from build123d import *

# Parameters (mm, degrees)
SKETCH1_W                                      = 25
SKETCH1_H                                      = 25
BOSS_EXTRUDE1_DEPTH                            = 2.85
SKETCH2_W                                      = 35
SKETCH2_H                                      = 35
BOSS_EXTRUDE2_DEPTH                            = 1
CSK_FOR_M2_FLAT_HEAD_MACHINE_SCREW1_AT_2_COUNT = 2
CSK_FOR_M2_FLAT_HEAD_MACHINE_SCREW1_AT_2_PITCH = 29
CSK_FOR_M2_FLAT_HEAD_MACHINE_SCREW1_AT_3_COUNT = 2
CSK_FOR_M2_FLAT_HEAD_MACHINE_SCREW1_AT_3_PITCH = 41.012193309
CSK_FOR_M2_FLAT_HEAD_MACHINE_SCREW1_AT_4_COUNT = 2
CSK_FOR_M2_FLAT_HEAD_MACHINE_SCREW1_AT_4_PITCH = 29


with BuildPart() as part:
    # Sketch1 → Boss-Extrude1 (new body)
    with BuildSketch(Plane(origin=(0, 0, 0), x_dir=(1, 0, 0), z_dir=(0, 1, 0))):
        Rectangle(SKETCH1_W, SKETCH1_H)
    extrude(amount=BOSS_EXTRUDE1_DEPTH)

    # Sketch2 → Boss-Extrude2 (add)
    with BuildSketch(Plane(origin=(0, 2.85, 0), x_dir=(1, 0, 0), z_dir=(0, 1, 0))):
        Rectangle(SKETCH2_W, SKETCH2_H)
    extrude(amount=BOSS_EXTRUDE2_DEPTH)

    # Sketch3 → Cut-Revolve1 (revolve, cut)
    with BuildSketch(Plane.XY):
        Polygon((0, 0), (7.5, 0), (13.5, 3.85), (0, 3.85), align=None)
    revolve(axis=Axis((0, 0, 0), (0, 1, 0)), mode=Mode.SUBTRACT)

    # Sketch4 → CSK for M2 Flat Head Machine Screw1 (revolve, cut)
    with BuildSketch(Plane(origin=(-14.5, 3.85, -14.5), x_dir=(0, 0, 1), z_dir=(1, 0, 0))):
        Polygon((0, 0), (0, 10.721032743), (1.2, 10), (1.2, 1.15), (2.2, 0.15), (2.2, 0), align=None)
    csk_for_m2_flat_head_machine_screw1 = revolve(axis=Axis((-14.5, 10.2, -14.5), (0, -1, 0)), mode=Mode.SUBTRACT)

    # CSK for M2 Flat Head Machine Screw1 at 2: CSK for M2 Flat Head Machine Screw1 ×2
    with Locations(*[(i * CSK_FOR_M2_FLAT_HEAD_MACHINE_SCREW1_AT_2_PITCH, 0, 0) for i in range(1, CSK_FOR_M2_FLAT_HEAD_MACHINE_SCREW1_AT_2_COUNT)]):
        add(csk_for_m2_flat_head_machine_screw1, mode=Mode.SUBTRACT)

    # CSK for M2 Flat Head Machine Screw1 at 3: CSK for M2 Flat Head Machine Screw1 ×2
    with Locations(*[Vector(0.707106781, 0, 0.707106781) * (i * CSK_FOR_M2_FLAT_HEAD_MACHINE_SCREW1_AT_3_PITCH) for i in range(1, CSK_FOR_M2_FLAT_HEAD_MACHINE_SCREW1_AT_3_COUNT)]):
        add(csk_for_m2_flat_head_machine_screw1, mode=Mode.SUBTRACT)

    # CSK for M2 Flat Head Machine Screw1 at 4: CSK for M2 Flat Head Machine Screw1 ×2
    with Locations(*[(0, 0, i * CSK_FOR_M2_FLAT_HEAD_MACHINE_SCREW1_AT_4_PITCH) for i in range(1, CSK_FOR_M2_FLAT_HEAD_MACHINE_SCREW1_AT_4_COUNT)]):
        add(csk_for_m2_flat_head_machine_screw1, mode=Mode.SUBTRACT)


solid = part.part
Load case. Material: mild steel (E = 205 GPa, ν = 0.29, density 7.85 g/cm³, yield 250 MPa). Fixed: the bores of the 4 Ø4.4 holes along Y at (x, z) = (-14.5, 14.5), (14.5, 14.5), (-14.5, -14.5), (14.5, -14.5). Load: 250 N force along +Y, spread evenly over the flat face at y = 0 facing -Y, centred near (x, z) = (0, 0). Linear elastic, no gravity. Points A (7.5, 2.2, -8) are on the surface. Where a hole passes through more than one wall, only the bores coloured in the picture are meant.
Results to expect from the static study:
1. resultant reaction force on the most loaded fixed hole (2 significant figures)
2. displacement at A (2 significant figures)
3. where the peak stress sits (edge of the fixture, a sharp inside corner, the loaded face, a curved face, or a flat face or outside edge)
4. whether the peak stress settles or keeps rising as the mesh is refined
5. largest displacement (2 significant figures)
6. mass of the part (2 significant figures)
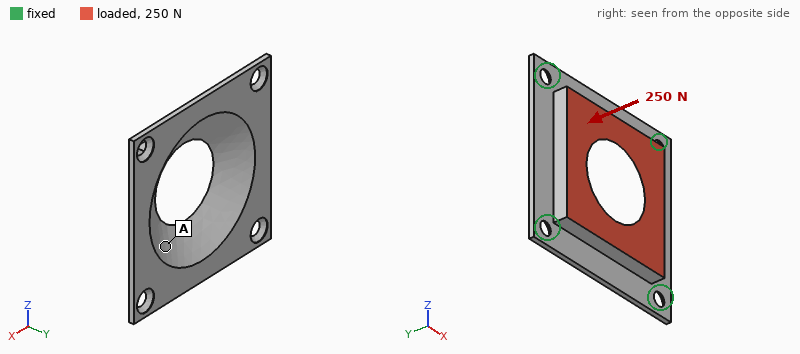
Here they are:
150 N
3.6 µm
edge of the fixture
keeps rising
5.1 µm
13 g
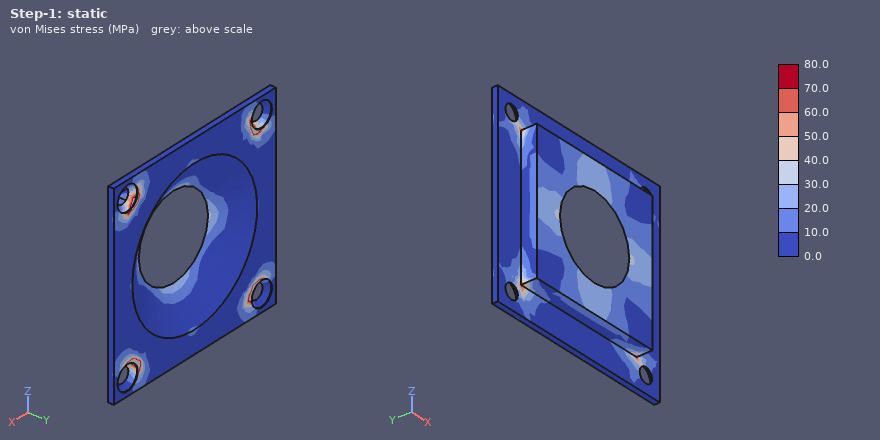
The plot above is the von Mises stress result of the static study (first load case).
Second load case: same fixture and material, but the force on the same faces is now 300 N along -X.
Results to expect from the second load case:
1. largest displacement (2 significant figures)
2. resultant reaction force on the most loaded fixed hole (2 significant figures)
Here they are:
1.5 µm
81 N
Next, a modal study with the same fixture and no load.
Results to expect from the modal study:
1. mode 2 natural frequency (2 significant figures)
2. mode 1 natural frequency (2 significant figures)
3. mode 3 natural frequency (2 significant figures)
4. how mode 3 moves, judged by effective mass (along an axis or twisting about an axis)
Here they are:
14 kHz
14 kHz
15 kHz
twisting about Z
